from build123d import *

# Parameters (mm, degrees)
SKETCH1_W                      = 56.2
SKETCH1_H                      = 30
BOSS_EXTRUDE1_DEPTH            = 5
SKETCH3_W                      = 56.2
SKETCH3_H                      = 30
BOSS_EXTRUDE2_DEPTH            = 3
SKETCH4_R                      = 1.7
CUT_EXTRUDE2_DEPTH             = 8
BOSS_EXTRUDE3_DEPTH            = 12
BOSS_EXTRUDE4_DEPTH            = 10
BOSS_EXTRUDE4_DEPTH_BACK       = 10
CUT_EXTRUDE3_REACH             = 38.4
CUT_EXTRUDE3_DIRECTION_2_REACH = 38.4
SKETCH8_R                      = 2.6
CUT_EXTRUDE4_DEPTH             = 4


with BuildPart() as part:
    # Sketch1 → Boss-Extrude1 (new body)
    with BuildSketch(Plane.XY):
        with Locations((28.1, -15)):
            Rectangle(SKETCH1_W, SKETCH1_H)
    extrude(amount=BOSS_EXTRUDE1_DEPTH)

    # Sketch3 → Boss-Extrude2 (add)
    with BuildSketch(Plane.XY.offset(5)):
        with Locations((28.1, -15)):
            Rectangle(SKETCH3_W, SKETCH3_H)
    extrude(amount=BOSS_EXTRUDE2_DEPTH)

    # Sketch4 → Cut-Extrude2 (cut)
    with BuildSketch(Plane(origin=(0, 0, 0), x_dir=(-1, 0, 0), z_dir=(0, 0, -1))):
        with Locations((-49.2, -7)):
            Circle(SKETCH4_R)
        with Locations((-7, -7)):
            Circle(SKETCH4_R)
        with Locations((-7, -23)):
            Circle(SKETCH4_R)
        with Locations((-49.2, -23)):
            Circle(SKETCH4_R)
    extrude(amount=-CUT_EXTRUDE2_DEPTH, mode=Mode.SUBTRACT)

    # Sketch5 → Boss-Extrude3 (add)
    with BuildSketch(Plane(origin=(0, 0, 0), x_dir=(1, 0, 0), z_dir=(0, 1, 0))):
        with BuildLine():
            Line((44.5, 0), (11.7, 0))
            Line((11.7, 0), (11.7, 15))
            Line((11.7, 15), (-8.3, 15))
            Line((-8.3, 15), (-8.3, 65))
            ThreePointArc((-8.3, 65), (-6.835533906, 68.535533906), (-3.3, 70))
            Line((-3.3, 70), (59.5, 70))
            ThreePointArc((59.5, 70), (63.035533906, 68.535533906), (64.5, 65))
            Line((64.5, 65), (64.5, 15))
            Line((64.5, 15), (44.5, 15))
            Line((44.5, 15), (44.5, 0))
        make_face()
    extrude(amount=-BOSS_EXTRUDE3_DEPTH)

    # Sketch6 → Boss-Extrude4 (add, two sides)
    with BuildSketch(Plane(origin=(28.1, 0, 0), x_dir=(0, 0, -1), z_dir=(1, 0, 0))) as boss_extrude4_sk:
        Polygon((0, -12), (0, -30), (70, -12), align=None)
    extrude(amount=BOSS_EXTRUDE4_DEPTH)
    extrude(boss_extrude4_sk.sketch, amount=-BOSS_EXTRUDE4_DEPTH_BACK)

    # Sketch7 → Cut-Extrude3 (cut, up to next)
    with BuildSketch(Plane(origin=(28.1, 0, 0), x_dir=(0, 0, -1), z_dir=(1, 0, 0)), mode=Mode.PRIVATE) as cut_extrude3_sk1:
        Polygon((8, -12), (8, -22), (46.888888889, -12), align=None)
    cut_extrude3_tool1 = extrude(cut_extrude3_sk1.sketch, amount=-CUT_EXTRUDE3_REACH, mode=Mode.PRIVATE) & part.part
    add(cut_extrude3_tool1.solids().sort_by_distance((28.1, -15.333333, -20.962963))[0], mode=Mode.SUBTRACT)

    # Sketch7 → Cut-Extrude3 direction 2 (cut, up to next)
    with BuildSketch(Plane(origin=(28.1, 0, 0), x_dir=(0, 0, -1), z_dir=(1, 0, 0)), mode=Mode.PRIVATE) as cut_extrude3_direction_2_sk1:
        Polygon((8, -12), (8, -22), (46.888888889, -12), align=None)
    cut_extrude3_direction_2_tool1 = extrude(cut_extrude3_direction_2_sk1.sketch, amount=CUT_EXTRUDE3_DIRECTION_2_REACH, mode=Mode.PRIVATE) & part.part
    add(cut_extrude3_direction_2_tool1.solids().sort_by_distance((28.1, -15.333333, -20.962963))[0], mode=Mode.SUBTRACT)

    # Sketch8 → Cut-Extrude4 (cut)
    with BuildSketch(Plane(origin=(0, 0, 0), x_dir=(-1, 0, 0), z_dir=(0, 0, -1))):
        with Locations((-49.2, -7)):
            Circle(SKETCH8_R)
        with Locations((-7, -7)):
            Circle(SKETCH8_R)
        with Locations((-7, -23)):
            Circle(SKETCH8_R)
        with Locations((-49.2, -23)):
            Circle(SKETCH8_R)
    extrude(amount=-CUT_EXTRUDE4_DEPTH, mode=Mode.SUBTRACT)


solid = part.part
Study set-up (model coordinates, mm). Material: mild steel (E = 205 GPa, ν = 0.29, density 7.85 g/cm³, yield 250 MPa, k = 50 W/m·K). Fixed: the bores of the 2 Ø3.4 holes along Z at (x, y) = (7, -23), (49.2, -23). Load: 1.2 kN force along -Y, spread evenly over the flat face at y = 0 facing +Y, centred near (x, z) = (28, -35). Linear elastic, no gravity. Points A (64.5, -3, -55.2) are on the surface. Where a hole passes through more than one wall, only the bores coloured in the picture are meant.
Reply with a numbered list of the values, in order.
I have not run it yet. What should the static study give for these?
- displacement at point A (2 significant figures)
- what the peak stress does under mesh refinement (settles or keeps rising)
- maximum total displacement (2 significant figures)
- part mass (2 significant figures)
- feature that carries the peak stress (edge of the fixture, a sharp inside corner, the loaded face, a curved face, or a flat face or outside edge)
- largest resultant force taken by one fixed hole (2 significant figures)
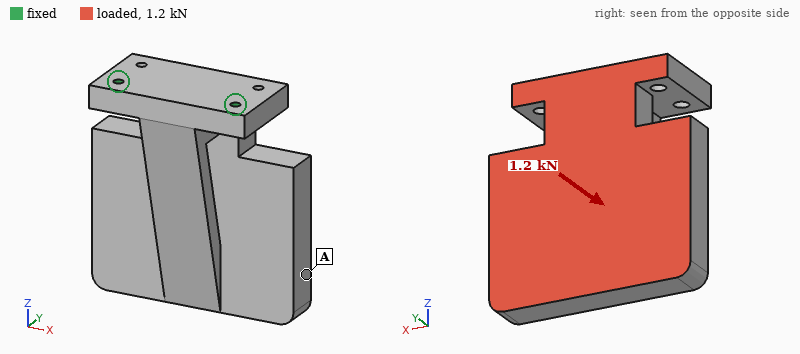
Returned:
1. 0.21 mm
2. keeps rising
3. 0.26 mm
4. 590 g
5. edge of the fixture
6. 900 N
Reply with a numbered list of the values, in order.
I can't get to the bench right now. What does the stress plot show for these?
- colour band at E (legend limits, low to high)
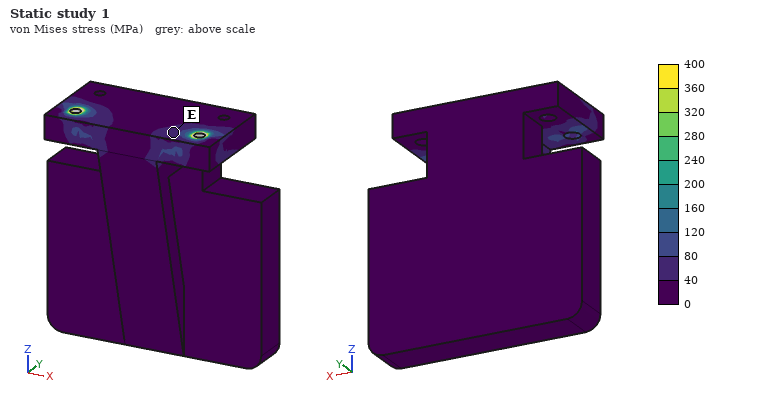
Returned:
1. 40 to 80 MPa
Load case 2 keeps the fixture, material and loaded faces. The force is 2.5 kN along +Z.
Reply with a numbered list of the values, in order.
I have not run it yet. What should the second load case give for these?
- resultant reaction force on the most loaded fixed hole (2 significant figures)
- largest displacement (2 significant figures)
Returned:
1. 1.3 kN
2. 0.29 mm
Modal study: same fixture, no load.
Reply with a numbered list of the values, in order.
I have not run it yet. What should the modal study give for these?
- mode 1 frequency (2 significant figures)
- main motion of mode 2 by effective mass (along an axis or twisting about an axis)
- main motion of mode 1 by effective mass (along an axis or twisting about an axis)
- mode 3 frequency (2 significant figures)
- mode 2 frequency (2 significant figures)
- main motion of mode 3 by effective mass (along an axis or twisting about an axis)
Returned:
1. 560 Hz
2. along X
3. along Y
4. 3000 Hz
5. 1600 Hz
6. twisting about Z
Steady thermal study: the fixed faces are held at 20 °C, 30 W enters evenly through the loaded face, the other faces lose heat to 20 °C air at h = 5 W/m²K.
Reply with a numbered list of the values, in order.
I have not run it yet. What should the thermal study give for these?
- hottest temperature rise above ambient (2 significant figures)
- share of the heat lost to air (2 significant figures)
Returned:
1. 63 K
2. 10 %
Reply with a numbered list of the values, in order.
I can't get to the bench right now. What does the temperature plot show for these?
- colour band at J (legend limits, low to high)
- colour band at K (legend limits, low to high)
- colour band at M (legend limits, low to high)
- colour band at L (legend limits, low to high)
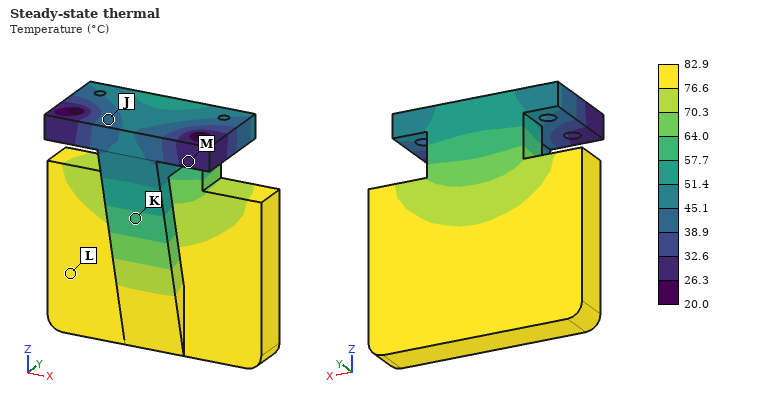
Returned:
1. 38.9 to 45.1 °C
2. 57.7 to 64.0 °C
3. 26.3 to 32.6 °C
4. 76.6 to 82.9 °C
